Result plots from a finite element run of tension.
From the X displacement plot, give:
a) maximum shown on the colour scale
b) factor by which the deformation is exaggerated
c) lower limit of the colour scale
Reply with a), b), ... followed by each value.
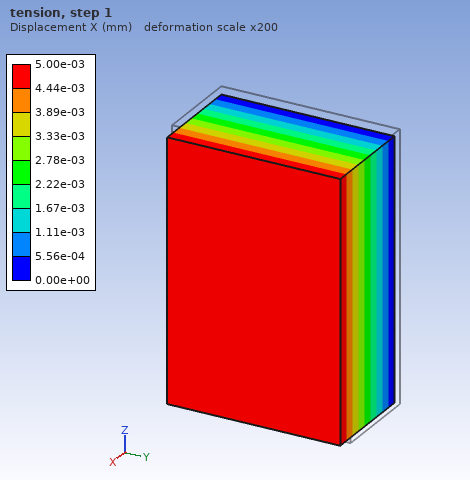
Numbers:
a) 5.00e-03 mm
b) 200
c) 0.00e+00 mm
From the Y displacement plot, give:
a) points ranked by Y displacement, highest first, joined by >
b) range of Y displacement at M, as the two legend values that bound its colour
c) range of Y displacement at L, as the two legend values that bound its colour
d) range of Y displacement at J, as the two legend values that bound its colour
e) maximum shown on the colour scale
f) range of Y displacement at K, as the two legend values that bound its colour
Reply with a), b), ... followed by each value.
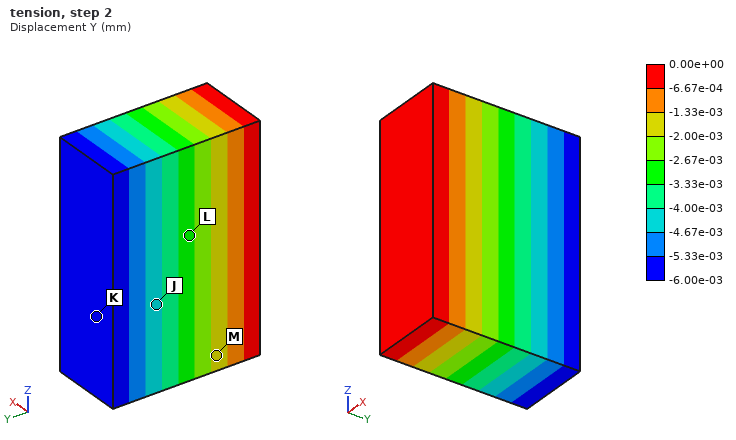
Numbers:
a) M > L > J > K
b) -2.00e-03 to -1.33e-03 mm
c) -3.33e-03 to -2.67e-03 mm
d) -4.67e-03 to -4.00e-03 mm
e) 0.00e+00 mm
f) -6.00e-03 to -5.33e-03 mm
